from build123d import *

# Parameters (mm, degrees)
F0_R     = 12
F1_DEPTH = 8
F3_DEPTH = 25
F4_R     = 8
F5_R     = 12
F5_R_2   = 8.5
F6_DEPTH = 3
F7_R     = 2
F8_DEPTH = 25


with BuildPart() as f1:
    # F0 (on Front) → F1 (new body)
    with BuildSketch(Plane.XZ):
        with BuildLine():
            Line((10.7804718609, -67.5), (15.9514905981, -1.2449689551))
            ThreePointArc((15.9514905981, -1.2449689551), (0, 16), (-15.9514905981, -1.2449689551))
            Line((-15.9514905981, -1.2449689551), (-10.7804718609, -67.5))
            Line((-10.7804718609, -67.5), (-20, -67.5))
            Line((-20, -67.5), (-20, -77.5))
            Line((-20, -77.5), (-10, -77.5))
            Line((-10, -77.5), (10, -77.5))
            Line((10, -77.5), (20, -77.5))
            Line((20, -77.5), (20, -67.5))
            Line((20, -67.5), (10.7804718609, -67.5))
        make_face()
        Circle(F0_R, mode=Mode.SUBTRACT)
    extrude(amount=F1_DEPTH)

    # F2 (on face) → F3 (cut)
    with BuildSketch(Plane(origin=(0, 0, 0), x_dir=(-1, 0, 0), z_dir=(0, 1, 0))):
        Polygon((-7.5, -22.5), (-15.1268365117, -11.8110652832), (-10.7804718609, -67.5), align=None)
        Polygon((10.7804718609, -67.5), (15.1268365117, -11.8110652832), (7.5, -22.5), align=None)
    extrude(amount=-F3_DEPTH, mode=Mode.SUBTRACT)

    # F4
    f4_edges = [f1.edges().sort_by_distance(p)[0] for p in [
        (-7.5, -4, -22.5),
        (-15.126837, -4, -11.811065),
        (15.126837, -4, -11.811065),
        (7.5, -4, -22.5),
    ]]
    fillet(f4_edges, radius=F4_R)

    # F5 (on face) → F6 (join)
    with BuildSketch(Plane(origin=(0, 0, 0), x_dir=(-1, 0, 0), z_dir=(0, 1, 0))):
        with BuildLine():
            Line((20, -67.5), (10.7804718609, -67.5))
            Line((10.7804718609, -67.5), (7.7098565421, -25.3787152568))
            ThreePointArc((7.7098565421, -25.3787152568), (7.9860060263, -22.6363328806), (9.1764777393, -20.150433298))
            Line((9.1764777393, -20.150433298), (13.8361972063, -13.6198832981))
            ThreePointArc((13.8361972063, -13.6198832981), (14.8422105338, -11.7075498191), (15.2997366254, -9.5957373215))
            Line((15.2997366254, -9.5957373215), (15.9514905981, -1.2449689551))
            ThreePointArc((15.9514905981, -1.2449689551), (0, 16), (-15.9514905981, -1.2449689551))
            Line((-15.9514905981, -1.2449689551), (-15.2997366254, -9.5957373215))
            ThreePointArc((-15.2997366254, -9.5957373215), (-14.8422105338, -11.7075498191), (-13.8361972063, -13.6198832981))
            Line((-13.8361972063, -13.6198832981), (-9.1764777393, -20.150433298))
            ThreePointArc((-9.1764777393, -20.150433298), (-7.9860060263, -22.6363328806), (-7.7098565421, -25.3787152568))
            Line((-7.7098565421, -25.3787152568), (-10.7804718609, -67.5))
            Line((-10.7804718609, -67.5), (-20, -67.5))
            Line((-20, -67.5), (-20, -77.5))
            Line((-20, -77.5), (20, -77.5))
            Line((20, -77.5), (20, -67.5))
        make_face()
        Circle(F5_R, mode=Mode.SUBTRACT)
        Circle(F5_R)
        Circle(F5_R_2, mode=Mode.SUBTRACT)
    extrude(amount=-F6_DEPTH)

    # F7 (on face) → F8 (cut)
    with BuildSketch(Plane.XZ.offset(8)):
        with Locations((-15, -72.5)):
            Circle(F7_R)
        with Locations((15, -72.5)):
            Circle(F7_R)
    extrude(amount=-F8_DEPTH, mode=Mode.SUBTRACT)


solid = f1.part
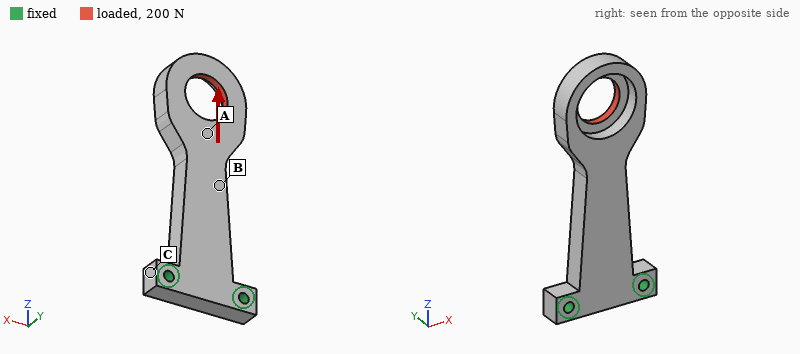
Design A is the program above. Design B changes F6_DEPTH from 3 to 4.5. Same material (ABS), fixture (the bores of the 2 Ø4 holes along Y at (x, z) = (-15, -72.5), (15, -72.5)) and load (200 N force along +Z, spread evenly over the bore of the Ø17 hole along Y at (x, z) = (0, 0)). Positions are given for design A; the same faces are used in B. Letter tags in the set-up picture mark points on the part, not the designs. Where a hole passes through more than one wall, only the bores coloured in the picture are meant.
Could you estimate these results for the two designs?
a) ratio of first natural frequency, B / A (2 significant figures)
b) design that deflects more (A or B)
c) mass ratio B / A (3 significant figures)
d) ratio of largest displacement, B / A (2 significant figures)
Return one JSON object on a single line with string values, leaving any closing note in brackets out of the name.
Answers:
{"ratio of first natural frequency, B / A": "0.97", "design that deflects more": "A", "mass ratio B / A": "1.02", "ratio of largest displacement, B / A": "0.69"}
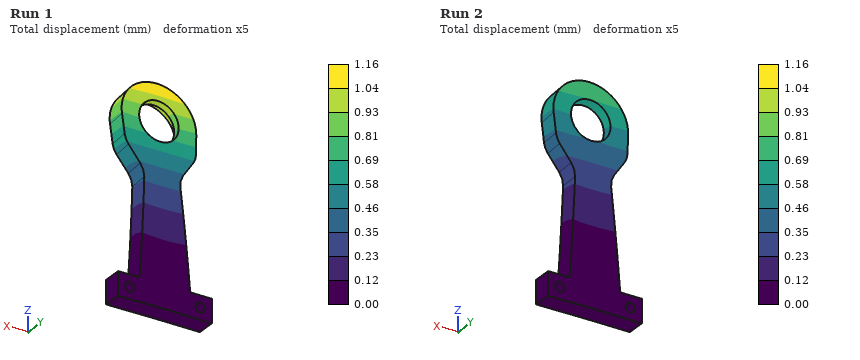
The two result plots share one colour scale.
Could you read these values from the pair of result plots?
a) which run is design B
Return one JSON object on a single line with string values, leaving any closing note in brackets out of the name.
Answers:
{"which run is design B": "Run 2"}
